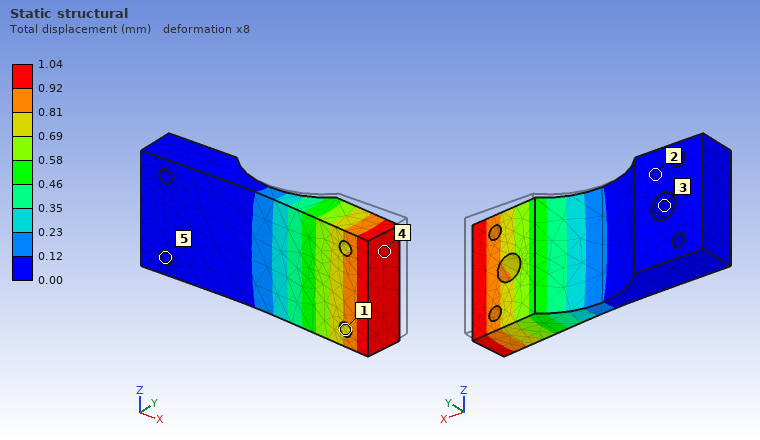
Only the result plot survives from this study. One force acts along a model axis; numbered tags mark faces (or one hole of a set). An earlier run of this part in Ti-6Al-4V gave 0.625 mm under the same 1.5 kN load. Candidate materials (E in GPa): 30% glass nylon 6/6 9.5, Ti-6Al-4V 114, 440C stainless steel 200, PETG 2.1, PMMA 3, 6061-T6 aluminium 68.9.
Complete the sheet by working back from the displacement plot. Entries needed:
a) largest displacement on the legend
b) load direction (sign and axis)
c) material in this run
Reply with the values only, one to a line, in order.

1.04 mm
-Y
6061-T6 aluminium
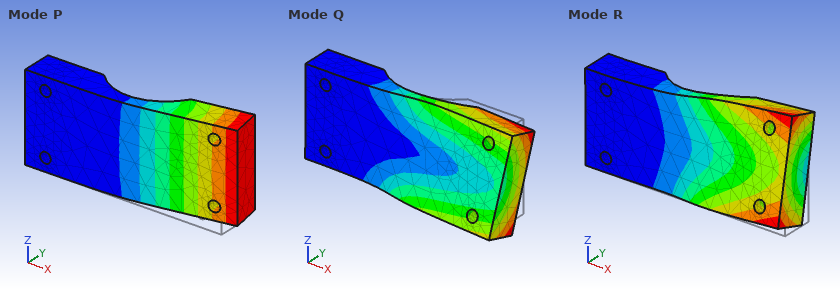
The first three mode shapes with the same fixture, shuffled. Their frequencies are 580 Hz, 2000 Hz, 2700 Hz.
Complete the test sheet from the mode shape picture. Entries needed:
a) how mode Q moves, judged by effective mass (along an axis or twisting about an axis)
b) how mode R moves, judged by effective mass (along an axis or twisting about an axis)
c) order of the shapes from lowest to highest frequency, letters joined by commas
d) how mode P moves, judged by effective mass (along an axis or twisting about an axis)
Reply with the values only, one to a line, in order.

along Z
along Z
P, Q, R
along Y
